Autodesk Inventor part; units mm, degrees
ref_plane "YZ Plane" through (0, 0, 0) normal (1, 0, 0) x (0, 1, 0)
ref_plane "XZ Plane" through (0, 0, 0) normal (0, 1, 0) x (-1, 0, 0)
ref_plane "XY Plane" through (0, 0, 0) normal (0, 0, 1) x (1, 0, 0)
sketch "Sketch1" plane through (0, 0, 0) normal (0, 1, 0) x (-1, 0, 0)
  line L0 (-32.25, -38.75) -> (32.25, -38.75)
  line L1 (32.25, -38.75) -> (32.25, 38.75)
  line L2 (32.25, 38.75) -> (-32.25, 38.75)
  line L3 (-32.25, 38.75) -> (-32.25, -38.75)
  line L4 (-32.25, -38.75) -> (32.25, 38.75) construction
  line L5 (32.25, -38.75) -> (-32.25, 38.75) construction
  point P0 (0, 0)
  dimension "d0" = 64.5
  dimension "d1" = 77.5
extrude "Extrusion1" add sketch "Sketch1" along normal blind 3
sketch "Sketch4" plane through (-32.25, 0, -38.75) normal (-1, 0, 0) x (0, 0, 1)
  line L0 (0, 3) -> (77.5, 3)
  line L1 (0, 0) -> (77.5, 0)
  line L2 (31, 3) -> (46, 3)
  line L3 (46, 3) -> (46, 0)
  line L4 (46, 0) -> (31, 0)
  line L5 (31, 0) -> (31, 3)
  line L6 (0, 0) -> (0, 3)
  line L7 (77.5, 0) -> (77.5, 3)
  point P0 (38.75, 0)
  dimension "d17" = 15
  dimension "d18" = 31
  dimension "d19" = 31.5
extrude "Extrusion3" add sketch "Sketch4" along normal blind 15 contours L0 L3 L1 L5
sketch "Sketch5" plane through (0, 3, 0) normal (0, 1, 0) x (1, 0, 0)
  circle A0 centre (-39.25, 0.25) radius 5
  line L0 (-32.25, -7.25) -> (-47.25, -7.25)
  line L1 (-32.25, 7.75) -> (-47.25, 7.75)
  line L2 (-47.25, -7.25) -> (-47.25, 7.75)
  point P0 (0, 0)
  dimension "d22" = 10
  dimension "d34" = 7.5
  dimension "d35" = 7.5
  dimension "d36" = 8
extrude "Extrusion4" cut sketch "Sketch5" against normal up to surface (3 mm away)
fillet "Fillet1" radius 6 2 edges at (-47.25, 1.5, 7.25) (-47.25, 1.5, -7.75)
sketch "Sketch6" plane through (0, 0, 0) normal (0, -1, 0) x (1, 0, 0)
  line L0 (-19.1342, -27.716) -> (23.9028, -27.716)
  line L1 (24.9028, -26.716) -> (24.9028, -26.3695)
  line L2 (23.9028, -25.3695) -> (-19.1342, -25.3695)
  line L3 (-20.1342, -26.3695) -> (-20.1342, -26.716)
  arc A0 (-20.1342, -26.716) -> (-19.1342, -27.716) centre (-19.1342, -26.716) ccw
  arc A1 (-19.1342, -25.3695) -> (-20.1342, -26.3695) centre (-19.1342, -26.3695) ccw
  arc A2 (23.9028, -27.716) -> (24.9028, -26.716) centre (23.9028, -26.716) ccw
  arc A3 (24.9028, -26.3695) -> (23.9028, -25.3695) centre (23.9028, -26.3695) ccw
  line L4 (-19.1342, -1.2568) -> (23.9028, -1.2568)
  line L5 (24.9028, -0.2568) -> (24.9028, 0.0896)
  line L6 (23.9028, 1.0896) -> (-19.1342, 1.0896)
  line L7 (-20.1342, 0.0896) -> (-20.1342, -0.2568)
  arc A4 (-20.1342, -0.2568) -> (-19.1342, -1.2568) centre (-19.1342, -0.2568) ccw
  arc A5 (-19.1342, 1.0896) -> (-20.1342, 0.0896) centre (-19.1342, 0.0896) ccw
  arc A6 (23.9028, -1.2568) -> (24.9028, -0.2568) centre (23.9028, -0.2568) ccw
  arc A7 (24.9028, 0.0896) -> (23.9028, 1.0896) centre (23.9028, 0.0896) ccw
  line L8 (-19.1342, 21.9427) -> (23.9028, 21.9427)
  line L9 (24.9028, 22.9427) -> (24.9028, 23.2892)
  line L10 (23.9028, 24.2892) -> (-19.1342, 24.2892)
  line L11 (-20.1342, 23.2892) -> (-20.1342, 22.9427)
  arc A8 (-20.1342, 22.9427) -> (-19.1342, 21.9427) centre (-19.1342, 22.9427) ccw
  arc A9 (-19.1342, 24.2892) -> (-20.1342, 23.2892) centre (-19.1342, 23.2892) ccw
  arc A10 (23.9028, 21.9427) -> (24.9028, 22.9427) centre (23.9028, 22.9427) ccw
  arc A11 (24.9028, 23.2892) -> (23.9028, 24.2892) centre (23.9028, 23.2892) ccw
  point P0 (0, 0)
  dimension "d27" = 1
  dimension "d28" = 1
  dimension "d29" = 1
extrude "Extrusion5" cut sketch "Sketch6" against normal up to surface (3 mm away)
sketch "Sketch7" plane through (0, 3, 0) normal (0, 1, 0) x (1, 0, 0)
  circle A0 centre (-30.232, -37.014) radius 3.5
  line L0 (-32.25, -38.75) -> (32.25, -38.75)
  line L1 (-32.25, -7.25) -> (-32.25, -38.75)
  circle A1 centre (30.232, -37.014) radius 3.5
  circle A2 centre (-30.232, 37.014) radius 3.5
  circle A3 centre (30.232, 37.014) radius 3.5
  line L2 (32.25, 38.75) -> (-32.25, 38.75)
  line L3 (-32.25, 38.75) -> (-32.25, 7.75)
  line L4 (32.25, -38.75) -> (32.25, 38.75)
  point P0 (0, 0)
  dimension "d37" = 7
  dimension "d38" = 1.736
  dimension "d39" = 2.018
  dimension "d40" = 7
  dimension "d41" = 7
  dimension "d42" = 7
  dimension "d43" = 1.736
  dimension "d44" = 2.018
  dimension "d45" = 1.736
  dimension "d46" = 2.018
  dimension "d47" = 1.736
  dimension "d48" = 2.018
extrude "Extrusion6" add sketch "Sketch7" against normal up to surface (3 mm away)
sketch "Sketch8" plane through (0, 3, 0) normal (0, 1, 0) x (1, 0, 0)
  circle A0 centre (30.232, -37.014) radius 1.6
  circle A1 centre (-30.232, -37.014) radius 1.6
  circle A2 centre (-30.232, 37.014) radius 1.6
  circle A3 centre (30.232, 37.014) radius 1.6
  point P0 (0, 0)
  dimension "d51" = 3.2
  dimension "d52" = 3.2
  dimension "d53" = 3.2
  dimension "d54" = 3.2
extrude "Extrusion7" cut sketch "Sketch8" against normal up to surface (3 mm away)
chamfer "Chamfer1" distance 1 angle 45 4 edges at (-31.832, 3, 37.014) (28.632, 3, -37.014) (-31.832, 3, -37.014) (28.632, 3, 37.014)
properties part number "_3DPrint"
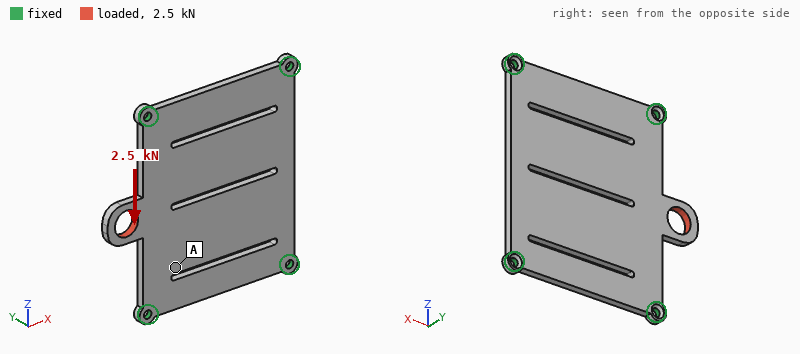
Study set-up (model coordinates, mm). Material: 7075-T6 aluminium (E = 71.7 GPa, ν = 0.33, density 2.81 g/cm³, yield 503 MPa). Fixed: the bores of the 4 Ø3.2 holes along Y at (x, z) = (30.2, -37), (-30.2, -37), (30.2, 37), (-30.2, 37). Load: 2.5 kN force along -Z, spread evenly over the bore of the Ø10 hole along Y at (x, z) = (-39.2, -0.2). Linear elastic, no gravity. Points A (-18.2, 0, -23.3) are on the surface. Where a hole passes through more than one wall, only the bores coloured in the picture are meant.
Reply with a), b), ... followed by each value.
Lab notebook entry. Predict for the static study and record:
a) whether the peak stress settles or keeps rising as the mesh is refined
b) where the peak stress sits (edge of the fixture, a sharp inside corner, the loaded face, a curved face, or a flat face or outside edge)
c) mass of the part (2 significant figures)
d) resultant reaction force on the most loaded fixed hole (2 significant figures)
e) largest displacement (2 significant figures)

a) keeps rising
b) a sharp inside corner
c) 41 g
d) 1.1 kN
e) 0.23 mm
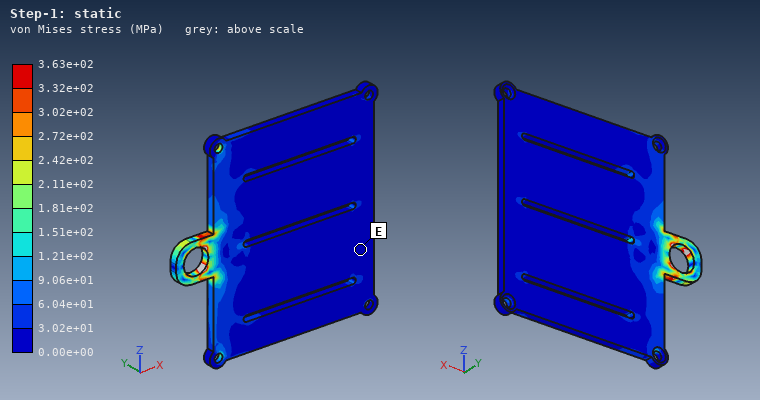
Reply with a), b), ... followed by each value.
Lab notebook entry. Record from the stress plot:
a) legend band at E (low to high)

a) 0.00e+00 to 3.02e+01 MPa
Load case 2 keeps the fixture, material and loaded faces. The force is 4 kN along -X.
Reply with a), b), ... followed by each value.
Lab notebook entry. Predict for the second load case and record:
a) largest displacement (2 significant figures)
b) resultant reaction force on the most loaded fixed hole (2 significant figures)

a) 0.11 mm
b) 1.3 kN
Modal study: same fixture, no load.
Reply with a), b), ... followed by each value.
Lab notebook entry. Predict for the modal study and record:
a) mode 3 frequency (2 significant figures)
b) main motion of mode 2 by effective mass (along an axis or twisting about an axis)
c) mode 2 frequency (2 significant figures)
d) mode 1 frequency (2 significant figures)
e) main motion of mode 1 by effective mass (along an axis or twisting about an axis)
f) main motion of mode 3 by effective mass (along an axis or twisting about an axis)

a) 3200 Hz
b) twisting about Z
c) 2600 Hz
d) 1500 Hz
e) along Y
f) twisting about X
